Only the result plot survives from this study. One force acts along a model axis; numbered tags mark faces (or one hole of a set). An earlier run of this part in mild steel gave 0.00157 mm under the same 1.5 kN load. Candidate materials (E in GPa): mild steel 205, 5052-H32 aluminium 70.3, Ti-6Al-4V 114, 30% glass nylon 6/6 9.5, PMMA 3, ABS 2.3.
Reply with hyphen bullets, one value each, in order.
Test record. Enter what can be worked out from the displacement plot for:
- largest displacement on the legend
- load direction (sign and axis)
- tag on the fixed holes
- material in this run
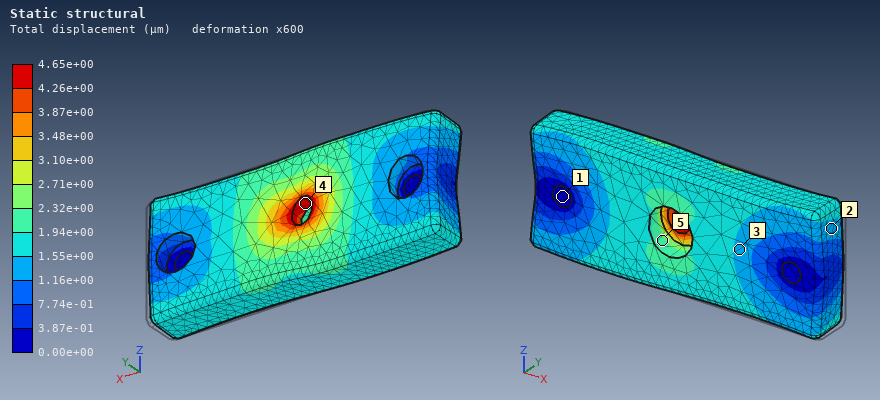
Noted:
- 4.65e+00 µm
- -X
- 1
- 5052-H32 aluminium
